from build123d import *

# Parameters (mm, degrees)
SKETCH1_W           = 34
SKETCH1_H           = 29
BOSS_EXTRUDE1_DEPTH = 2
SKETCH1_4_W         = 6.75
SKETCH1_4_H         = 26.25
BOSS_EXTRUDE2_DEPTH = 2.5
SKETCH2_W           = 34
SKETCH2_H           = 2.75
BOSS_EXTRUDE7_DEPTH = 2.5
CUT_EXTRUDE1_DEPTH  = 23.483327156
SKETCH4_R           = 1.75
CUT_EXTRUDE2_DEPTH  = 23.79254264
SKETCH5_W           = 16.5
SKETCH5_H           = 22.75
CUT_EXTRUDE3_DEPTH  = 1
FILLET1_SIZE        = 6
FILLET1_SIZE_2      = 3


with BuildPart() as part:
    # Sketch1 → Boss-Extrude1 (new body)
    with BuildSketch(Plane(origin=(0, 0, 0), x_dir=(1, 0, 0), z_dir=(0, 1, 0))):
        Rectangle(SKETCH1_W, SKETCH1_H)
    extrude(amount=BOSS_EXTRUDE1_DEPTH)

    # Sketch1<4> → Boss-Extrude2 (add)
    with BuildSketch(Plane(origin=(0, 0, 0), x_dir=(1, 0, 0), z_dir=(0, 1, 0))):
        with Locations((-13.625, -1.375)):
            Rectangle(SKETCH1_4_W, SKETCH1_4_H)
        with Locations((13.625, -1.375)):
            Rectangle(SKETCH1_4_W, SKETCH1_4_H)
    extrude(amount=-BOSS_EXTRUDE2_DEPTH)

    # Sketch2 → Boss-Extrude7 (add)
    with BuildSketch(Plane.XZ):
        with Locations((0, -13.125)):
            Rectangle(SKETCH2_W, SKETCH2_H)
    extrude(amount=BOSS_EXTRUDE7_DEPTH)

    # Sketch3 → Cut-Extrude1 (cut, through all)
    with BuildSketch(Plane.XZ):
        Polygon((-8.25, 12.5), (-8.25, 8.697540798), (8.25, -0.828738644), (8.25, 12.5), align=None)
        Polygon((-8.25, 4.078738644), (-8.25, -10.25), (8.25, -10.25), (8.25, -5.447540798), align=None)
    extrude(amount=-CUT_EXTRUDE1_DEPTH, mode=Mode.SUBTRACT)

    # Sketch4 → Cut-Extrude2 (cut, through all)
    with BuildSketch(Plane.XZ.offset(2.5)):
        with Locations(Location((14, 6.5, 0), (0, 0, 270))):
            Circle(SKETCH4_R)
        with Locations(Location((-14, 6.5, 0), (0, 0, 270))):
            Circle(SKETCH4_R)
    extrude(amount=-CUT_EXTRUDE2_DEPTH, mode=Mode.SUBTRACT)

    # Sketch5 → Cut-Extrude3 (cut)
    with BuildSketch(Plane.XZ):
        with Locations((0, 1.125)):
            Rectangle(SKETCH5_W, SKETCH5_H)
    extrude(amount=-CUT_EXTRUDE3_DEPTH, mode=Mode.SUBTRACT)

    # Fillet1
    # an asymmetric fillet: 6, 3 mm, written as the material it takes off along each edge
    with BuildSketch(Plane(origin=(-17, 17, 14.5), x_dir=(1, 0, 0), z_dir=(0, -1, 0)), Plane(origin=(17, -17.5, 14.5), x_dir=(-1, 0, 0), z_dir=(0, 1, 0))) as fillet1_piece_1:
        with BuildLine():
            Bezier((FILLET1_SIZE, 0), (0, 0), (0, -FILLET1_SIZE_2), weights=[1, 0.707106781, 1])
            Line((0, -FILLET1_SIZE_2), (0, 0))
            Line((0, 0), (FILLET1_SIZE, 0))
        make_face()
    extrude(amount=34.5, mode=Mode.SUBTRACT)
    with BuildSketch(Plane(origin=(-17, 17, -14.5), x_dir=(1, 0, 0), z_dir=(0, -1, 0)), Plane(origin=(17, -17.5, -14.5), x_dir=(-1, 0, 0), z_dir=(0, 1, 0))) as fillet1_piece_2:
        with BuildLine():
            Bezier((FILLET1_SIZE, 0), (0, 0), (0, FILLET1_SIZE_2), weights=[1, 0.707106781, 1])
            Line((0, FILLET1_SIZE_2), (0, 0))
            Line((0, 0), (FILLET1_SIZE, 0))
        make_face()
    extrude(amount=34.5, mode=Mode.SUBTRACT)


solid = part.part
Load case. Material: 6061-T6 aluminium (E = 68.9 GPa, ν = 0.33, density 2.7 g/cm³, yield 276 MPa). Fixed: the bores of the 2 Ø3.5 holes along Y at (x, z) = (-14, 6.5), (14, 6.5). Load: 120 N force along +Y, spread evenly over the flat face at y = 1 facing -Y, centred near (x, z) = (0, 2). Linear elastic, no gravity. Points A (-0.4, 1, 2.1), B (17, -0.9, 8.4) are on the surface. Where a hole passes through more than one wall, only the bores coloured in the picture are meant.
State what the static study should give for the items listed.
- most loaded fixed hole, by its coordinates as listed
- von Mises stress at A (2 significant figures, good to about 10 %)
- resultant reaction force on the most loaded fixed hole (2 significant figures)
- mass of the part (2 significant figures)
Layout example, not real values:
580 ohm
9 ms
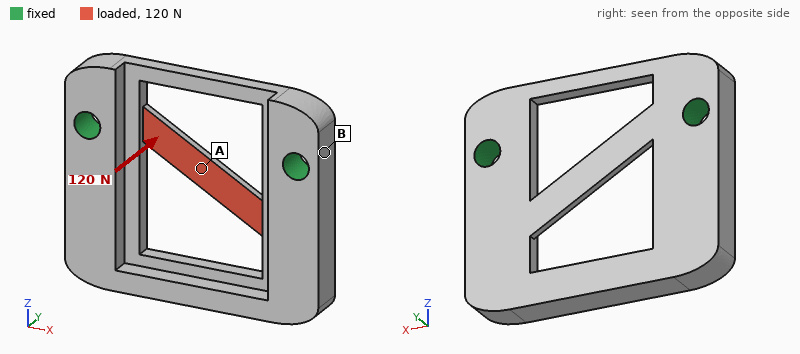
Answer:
(-14, 6.5)
130 MPa
70 N
6.1 g
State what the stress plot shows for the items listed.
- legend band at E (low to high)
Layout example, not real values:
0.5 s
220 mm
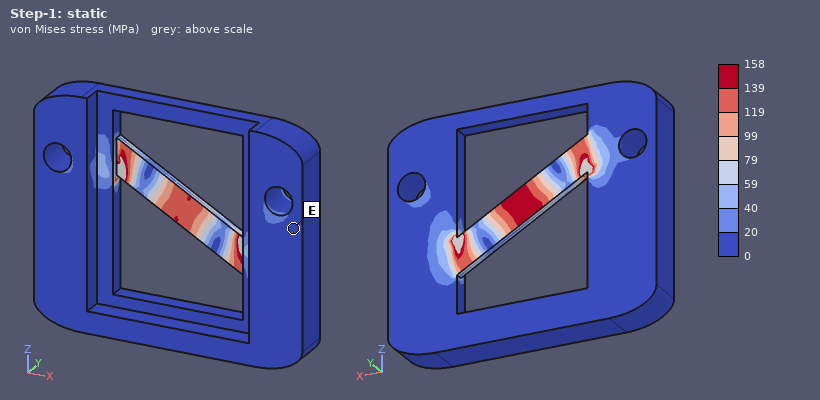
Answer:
0 to 20 MPa
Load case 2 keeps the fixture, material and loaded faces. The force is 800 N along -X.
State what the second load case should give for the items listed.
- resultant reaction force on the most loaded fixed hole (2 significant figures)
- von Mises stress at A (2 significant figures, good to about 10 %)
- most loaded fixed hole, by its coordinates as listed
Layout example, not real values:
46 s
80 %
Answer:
500 N
44 MPa
(-14, 6.5)
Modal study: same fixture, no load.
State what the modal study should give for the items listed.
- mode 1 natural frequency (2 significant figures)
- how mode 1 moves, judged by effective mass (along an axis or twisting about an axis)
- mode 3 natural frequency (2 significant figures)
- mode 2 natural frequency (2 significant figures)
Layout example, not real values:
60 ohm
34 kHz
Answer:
6800 Hz
along Y
13 kHz
11 kHz
